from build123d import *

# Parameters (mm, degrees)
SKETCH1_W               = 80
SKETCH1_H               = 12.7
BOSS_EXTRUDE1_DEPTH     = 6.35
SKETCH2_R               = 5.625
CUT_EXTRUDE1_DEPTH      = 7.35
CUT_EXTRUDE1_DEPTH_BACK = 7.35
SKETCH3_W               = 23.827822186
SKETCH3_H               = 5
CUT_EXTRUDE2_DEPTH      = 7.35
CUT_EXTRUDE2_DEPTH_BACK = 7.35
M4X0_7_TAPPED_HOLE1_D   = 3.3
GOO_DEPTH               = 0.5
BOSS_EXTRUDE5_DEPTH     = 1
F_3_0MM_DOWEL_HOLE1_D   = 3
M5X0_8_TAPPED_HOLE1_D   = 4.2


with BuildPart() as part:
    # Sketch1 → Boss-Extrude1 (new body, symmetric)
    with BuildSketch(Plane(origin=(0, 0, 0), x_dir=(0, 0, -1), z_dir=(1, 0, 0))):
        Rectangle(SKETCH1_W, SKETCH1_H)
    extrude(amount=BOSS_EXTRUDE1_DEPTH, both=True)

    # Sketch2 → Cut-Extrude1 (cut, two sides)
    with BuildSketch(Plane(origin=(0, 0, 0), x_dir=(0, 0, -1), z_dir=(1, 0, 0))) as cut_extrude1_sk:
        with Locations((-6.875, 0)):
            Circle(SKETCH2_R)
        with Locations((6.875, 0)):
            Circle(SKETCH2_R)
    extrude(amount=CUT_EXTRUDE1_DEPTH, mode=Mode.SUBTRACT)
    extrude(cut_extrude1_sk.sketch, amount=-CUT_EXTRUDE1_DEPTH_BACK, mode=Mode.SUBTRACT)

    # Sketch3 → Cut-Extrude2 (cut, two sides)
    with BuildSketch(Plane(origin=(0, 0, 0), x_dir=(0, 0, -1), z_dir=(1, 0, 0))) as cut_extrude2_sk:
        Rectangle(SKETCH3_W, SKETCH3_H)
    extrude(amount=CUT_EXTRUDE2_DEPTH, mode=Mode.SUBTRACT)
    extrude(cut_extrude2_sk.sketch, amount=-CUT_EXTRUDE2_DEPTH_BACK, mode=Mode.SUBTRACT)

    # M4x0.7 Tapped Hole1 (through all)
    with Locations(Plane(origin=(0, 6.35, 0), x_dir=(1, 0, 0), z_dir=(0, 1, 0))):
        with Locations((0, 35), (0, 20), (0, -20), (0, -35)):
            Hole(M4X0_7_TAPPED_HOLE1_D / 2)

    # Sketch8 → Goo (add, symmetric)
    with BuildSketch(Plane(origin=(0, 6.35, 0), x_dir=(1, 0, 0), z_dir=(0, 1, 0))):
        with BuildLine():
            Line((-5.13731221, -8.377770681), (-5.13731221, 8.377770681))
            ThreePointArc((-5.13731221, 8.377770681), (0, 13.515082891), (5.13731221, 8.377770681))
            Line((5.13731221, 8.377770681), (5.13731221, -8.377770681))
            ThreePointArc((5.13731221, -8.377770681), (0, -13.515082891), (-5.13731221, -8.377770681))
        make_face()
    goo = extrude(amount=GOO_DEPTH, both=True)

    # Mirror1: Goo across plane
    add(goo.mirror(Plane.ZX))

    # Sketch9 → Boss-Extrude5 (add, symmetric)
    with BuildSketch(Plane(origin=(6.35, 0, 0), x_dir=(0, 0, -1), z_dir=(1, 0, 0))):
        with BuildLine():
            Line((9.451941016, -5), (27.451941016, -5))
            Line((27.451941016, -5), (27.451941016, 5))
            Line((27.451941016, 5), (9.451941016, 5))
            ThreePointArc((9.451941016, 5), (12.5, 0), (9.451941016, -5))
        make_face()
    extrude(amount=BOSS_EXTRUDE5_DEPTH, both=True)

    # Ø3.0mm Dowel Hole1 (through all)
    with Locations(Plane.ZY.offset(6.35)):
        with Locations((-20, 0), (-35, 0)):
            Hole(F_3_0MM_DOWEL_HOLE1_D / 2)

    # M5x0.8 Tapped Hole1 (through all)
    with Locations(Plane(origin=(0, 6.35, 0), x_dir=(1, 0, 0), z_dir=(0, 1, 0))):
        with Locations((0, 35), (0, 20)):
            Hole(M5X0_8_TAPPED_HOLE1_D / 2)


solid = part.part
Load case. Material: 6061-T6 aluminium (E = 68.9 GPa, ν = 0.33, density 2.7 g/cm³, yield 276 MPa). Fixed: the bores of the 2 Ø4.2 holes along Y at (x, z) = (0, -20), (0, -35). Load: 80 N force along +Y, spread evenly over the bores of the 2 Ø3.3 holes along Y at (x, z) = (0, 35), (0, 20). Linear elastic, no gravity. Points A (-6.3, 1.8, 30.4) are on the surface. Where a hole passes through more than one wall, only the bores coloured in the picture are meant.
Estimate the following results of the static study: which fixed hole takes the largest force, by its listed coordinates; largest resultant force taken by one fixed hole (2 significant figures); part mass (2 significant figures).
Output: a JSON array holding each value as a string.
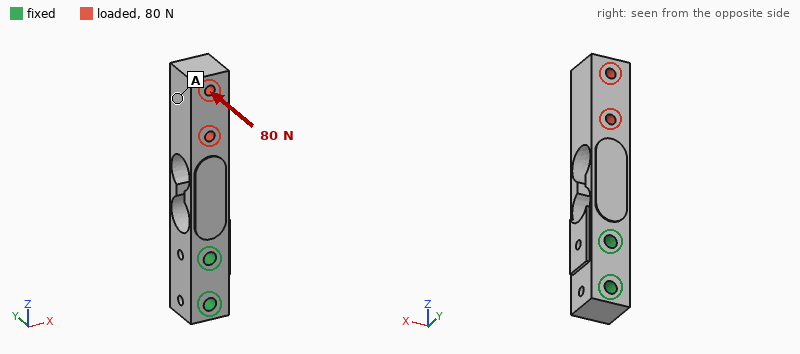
["(0, -20)", "110 N", "27 g"]
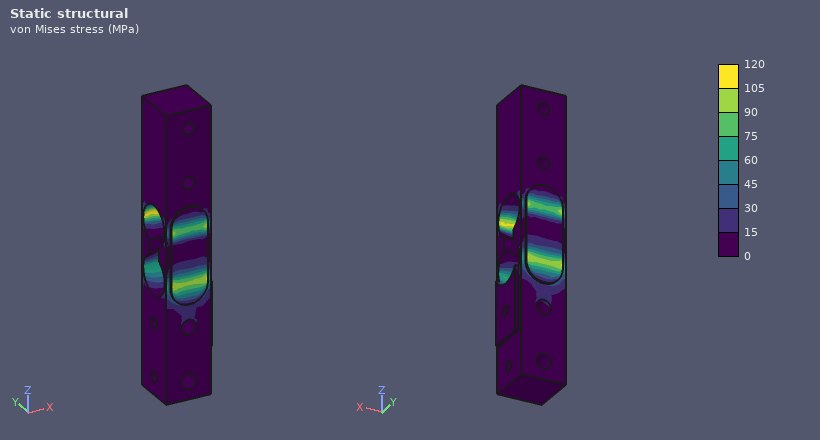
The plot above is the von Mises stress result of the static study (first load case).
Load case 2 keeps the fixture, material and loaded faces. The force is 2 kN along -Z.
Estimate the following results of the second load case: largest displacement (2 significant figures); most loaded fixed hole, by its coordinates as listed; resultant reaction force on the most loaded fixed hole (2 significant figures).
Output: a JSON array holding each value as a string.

["30 µm", "(0, -20)", "1.8 kN"]
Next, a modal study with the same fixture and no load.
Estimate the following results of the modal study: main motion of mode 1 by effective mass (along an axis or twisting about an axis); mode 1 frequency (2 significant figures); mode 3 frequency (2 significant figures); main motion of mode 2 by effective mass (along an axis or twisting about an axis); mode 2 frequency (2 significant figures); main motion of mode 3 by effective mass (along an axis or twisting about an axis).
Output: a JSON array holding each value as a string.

["along Y", "940 Hz", "5600 Hz", "along X", "1500 Hz", "twisting about Z"]
